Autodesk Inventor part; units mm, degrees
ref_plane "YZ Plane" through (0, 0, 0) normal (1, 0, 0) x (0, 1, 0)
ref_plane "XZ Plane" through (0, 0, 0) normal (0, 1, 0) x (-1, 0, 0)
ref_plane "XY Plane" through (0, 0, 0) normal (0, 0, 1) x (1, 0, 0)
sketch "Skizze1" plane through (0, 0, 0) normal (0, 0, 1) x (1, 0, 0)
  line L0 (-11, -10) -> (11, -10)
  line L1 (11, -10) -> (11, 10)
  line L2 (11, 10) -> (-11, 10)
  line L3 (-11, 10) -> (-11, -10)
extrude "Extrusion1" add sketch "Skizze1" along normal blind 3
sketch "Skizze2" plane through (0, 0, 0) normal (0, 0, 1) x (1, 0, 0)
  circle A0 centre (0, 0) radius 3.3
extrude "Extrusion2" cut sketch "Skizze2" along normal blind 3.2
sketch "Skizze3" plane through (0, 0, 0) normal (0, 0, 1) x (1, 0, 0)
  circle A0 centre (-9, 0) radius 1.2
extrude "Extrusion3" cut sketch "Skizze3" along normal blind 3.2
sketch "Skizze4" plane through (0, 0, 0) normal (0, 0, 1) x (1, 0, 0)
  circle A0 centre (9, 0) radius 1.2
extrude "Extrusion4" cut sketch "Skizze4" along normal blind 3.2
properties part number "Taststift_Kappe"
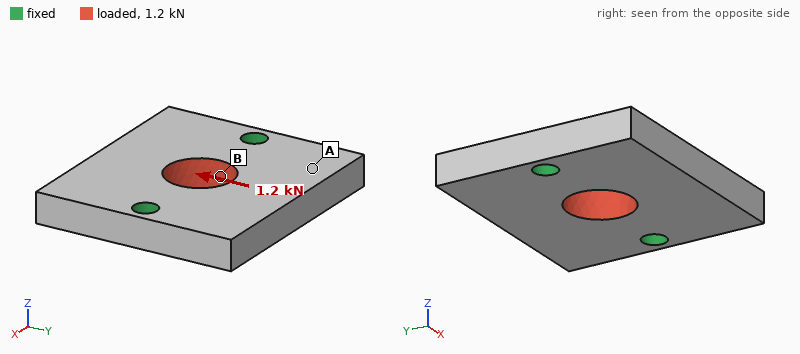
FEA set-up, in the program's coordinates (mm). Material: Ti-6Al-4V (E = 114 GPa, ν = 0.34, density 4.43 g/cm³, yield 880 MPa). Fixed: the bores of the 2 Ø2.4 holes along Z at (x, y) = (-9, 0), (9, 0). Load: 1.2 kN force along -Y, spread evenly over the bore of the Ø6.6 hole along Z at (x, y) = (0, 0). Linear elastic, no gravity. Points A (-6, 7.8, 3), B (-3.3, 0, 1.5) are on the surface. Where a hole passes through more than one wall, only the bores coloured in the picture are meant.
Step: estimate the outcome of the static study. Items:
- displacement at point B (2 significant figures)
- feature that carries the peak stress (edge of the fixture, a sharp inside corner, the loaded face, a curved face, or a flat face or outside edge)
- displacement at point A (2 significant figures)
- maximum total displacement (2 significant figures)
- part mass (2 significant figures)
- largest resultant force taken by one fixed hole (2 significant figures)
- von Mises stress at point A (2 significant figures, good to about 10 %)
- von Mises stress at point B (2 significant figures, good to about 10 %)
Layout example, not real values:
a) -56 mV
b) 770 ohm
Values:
a) 2.4 µm
b) edge of the fixture
c) 1.5 µm
d) 3.0 µm
e) 5.3 g
f) 600 N
g) 12 MPa
h) 33 MPa
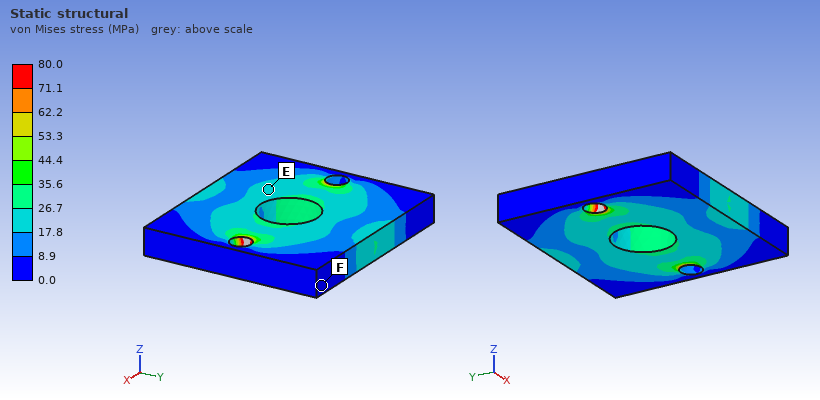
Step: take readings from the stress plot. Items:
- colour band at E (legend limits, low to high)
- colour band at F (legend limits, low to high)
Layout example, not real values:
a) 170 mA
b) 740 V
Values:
a) 17.8 to 26.7 MPa
b) 0.0 to 8.9 MPa
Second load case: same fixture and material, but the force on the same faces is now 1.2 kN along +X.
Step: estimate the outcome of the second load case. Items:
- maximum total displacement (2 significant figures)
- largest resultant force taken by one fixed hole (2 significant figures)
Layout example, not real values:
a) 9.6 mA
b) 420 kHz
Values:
a) 2.1 µm
b) 600 N
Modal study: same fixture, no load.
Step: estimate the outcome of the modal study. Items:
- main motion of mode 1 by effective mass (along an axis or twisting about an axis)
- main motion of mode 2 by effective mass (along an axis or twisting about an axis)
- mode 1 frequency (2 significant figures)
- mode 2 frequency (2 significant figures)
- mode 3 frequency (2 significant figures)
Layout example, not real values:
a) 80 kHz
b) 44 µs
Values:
a) twisting about X
b) along Z
c) 17 kHz
d) 21 kHz
e) 32 kHz
